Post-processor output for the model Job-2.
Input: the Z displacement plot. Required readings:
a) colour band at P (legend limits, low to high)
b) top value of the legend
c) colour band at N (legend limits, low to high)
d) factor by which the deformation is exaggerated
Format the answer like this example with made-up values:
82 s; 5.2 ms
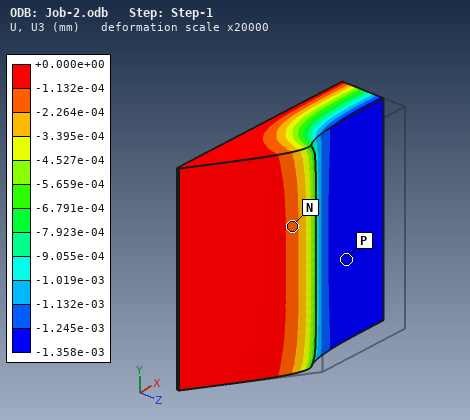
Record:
-1.358e-03 to -1.245e-03 mm; +0.000e+00 mm; -2.264e-04 to -1.132e-04 mm; 20000
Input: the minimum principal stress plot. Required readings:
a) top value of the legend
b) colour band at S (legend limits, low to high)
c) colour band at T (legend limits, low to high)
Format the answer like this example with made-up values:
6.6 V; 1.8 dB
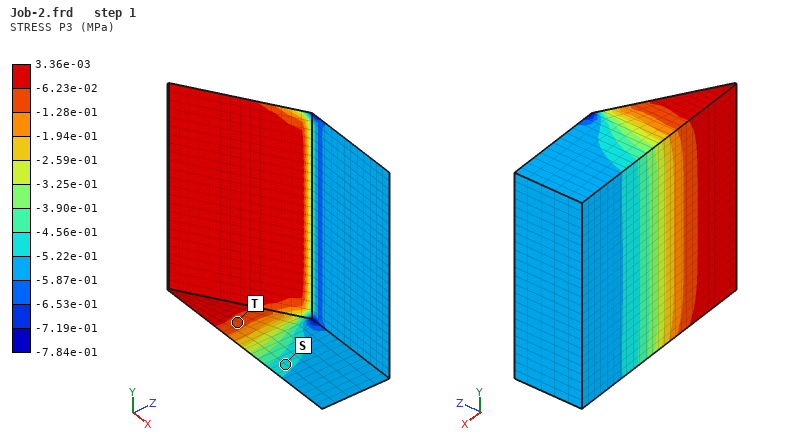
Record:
3.36e-03 MPa; -5.22e-01 to -4.56e-01 MPa; -1.28e-01 to -6.23e-02 MPa
